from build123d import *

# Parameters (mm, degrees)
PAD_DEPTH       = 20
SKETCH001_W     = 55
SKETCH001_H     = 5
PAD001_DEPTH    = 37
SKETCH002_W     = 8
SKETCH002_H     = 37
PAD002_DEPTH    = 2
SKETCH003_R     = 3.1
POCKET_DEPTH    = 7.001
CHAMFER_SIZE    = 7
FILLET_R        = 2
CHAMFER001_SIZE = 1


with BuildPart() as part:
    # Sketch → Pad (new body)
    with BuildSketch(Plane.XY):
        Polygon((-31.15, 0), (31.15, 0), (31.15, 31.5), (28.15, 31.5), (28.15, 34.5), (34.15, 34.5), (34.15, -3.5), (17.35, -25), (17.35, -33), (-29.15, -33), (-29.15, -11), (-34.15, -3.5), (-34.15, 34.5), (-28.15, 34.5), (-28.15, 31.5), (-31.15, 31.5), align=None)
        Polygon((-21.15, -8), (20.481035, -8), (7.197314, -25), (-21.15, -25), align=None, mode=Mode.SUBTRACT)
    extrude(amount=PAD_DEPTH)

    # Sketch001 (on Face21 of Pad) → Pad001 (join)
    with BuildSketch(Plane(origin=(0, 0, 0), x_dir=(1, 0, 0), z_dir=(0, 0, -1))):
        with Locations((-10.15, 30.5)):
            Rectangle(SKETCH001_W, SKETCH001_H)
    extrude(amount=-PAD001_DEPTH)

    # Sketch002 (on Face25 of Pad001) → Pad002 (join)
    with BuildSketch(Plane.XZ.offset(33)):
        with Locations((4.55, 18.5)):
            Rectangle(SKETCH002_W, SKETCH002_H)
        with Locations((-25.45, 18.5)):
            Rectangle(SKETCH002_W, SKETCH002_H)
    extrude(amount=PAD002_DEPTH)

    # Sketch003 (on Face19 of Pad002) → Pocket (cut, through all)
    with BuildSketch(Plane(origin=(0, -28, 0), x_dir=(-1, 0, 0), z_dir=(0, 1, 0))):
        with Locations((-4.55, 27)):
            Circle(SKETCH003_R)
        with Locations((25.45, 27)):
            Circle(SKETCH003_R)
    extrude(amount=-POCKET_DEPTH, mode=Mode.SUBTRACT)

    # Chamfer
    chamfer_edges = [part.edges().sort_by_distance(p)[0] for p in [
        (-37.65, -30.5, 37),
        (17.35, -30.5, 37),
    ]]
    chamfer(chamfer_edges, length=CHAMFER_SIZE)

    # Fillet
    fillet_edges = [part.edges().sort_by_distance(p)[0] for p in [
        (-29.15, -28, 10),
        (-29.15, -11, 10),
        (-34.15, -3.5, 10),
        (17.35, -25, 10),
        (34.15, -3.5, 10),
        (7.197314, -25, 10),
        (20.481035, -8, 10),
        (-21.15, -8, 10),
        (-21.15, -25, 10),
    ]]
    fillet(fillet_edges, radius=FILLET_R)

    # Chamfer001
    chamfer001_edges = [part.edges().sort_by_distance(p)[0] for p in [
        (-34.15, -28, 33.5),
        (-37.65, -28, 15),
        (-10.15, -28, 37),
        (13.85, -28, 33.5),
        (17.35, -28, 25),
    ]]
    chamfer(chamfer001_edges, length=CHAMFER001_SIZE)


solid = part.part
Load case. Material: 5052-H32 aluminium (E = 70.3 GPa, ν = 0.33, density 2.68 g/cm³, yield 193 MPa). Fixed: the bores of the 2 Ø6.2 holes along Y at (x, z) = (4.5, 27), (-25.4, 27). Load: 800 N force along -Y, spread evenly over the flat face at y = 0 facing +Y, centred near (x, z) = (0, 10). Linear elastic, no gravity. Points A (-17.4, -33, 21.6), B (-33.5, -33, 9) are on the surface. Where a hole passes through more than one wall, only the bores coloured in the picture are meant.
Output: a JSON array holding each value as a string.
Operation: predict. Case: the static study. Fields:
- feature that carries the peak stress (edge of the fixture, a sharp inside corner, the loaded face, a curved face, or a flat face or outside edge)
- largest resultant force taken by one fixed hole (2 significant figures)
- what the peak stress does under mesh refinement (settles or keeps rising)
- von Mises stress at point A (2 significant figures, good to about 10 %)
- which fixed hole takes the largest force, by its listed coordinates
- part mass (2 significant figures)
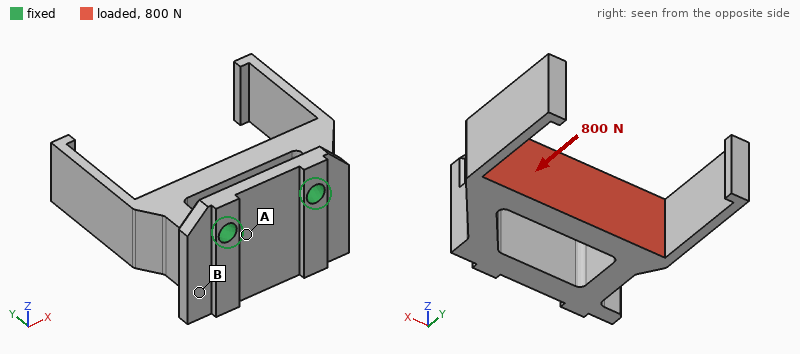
["edge of the fixture", "610 N", "keeps rising", "15 MPa", "(4.5, 27)", "94 g"]
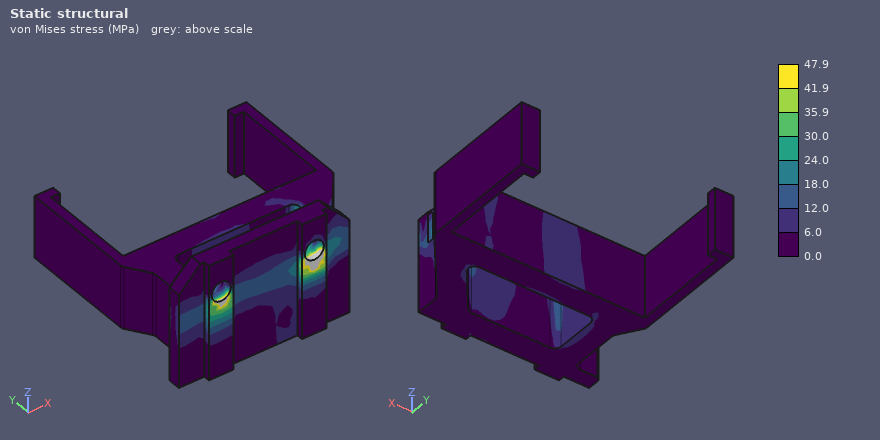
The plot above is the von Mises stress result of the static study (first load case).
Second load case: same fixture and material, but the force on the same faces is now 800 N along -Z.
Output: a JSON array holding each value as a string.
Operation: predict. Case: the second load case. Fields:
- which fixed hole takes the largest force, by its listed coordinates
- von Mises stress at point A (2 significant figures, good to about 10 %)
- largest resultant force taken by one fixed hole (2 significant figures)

["(4.5, 27)", "47 MPa", "630 N"]
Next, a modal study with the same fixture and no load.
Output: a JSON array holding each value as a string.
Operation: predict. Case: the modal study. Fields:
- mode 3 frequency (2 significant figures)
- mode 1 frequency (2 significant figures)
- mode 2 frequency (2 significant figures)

["1700 Hz", "1500 Hz", "1500 Hz"]
